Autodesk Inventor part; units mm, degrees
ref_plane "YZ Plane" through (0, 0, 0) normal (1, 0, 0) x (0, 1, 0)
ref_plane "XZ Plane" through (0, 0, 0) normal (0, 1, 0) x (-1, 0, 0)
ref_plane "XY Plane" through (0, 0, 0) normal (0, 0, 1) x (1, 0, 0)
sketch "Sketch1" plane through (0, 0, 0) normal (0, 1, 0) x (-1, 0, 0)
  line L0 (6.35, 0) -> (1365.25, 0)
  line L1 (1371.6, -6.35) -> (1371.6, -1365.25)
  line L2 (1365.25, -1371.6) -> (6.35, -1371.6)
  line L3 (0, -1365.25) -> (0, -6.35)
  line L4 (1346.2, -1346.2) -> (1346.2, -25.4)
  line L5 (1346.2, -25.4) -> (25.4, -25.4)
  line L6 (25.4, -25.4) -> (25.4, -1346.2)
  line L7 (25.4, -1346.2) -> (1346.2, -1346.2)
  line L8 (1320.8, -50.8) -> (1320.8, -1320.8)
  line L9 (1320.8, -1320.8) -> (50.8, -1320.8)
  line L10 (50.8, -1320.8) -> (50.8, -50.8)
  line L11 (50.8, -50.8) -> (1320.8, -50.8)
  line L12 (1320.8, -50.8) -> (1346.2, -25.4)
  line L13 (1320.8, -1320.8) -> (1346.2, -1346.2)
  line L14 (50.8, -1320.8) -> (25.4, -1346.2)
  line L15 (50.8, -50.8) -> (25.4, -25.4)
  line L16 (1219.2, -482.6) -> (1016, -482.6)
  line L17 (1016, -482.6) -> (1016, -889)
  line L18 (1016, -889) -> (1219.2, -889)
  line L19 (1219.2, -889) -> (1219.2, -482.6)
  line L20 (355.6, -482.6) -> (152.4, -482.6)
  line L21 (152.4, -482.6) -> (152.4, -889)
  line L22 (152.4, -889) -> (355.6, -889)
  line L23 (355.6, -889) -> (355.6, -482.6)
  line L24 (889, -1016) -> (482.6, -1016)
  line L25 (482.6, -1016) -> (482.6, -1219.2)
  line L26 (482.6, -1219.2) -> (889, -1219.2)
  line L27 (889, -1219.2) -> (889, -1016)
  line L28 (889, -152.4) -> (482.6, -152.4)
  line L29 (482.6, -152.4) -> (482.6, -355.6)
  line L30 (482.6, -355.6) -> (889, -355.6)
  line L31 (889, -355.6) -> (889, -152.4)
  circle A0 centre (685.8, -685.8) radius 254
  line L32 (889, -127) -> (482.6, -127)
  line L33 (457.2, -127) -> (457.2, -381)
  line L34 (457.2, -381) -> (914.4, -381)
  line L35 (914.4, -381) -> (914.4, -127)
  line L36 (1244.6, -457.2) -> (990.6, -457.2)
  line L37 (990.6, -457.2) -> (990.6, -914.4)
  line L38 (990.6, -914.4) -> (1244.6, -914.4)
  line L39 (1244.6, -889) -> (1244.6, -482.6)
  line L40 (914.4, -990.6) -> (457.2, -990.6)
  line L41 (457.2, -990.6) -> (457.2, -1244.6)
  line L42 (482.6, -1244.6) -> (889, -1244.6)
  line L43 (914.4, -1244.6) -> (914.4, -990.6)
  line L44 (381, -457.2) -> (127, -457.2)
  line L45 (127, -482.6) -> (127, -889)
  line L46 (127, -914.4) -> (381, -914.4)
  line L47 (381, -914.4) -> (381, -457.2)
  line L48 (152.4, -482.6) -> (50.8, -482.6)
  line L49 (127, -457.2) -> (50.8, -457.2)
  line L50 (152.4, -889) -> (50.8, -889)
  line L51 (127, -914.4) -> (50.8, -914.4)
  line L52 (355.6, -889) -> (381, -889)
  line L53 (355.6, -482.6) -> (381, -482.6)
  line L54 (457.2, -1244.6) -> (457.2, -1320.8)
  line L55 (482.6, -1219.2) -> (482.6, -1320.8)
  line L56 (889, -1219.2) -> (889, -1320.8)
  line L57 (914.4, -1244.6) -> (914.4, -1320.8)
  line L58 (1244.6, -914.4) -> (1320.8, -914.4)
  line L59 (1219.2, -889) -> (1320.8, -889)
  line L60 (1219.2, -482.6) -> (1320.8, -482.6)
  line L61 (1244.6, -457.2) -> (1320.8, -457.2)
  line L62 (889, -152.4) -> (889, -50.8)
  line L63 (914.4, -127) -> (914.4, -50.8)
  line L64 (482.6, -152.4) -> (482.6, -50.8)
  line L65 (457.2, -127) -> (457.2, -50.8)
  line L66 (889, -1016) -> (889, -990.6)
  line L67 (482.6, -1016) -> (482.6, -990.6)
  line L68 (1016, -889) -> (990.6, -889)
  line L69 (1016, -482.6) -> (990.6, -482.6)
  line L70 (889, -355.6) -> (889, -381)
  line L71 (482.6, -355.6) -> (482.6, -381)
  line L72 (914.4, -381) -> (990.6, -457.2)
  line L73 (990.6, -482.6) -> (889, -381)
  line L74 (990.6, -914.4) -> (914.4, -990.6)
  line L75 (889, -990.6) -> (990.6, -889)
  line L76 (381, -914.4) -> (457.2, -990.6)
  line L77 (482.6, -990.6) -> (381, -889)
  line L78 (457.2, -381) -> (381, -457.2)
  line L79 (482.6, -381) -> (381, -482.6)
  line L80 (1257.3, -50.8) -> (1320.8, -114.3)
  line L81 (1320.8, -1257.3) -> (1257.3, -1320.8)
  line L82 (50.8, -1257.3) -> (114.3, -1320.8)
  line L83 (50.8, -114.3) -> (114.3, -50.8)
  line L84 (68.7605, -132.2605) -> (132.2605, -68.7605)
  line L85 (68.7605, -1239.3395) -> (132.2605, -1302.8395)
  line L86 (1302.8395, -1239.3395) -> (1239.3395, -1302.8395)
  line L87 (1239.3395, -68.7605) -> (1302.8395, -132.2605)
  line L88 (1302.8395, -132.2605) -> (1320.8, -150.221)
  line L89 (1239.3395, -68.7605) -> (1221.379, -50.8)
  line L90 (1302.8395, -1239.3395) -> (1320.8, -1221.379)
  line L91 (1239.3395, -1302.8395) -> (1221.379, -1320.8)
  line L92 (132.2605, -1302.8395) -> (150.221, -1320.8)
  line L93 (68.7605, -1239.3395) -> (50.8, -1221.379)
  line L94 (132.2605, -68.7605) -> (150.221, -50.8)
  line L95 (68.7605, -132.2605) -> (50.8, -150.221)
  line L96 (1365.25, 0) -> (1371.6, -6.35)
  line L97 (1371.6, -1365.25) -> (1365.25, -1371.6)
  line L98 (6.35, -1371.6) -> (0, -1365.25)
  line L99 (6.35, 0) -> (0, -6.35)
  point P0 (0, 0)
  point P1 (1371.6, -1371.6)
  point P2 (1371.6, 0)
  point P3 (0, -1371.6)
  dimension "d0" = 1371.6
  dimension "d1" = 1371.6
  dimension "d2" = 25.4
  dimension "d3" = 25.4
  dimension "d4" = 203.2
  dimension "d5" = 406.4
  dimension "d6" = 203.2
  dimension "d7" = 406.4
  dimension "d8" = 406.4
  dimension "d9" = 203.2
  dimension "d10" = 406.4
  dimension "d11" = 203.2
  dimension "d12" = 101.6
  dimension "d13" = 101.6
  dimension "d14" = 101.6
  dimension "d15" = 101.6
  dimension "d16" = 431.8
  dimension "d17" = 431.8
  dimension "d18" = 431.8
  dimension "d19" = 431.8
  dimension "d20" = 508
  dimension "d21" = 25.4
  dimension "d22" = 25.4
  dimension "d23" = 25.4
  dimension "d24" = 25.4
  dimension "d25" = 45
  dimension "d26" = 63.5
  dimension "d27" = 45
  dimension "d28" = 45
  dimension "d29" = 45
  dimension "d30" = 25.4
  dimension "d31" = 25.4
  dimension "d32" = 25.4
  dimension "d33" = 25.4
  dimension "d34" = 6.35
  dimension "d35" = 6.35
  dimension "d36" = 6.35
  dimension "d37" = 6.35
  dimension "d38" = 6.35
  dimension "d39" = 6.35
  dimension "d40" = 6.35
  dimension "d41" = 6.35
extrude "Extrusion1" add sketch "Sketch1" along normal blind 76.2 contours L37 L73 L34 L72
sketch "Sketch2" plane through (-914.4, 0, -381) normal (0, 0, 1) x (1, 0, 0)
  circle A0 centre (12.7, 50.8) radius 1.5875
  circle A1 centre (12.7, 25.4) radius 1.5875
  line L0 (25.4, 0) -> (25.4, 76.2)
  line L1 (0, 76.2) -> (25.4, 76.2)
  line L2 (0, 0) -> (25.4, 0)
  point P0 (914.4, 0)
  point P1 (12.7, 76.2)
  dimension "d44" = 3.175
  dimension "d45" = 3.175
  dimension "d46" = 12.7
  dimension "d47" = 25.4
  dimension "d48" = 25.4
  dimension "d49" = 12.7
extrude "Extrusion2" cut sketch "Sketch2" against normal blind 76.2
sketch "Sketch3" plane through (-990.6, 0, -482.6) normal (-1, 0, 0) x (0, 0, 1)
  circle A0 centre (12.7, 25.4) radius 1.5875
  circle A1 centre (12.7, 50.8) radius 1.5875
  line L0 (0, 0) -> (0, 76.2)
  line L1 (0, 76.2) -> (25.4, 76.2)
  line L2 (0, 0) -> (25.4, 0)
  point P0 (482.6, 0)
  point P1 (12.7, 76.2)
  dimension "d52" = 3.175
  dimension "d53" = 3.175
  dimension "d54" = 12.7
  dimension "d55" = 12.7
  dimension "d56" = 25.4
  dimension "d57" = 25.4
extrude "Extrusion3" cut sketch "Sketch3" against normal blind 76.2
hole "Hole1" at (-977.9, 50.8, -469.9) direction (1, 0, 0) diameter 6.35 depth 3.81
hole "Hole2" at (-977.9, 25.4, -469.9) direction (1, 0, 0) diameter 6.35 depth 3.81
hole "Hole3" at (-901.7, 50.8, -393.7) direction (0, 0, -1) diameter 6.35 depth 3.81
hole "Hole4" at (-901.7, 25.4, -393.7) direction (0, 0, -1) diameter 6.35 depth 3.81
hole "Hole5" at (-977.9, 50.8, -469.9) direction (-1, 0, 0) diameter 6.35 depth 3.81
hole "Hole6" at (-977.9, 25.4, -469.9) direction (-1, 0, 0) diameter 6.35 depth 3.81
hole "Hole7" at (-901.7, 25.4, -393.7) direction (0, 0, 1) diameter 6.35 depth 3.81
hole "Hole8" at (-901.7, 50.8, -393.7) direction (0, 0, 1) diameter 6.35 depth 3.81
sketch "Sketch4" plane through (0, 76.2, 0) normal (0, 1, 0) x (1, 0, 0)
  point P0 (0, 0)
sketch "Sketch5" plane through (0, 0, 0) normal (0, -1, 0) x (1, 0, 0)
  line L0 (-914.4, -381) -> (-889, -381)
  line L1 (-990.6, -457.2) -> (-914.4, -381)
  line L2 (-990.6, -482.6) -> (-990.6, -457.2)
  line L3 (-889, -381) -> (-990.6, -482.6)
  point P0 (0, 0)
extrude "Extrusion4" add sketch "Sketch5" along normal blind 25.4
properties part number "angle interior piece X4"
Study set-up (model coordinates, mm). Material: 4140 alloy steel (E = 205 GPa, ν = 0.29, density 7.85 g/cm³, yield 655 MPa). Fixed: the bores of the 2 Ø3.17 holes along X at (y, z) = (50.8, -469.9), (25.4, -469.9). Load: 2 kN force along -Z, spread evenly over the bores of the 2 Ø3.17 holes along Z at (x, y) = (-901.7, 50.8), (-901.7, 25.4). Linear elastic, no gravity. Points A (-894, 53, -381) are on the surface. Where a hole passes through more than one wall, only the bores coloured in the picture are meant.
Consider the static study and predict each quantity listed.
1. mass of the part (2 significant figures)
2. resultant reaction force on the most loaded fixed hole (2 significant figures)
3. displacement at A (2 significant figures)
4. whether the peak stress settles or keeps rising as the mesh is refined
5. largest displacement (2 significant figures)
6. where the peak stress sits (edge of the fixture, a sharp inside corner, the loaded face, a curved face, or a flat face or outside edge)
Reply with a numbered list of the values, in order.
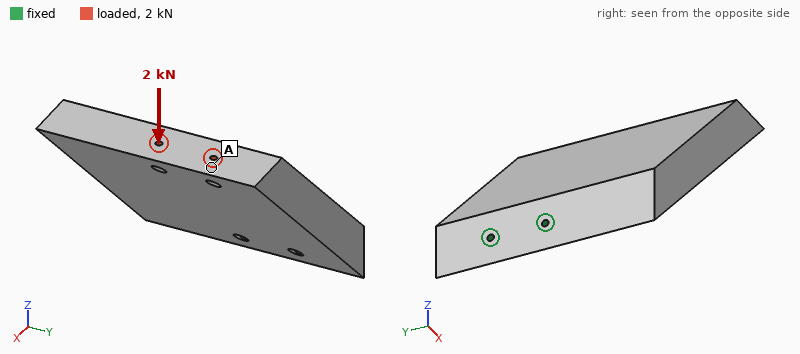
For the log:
1. 1.8 kg
2. 1.0 kN
3. 0.38 mm
4. keeps rising
5. 0.39 mm
6. edge of the fixture
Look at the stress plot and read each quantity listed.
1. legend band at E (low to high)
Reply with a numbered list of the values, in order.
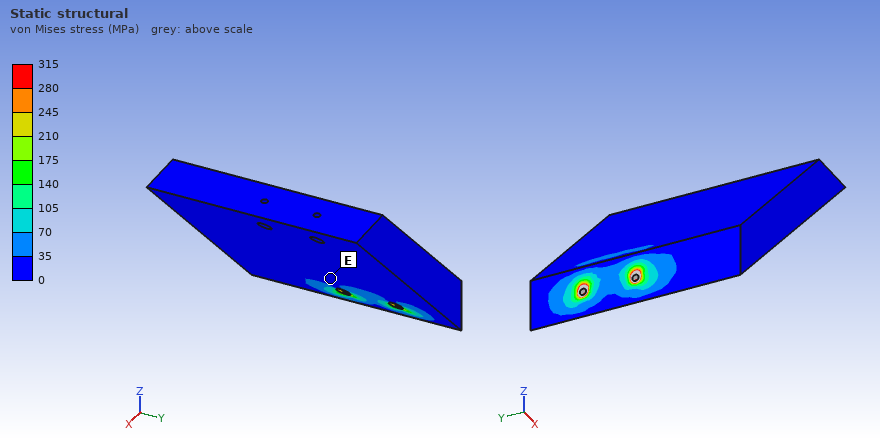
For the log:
1. 0 to 35 MPa
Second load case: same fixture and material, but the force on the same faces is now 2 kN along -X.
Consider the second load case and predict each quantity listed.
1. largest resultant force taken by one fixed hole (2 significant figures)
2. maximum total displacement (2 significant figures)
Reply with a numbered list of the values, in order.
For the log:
1. 1.0 kN
2. 0.38 mm
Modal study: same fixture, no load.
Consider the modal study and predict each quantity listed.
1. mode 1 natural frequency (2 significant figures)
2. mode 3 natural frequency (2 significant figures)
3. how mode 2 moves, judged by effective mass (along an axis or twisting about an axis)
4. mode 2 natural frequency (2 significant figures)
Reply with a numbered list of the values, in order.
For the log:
1. 420 Hz
2. 1600 Hz
3. along Y
4. 1200 Hz
